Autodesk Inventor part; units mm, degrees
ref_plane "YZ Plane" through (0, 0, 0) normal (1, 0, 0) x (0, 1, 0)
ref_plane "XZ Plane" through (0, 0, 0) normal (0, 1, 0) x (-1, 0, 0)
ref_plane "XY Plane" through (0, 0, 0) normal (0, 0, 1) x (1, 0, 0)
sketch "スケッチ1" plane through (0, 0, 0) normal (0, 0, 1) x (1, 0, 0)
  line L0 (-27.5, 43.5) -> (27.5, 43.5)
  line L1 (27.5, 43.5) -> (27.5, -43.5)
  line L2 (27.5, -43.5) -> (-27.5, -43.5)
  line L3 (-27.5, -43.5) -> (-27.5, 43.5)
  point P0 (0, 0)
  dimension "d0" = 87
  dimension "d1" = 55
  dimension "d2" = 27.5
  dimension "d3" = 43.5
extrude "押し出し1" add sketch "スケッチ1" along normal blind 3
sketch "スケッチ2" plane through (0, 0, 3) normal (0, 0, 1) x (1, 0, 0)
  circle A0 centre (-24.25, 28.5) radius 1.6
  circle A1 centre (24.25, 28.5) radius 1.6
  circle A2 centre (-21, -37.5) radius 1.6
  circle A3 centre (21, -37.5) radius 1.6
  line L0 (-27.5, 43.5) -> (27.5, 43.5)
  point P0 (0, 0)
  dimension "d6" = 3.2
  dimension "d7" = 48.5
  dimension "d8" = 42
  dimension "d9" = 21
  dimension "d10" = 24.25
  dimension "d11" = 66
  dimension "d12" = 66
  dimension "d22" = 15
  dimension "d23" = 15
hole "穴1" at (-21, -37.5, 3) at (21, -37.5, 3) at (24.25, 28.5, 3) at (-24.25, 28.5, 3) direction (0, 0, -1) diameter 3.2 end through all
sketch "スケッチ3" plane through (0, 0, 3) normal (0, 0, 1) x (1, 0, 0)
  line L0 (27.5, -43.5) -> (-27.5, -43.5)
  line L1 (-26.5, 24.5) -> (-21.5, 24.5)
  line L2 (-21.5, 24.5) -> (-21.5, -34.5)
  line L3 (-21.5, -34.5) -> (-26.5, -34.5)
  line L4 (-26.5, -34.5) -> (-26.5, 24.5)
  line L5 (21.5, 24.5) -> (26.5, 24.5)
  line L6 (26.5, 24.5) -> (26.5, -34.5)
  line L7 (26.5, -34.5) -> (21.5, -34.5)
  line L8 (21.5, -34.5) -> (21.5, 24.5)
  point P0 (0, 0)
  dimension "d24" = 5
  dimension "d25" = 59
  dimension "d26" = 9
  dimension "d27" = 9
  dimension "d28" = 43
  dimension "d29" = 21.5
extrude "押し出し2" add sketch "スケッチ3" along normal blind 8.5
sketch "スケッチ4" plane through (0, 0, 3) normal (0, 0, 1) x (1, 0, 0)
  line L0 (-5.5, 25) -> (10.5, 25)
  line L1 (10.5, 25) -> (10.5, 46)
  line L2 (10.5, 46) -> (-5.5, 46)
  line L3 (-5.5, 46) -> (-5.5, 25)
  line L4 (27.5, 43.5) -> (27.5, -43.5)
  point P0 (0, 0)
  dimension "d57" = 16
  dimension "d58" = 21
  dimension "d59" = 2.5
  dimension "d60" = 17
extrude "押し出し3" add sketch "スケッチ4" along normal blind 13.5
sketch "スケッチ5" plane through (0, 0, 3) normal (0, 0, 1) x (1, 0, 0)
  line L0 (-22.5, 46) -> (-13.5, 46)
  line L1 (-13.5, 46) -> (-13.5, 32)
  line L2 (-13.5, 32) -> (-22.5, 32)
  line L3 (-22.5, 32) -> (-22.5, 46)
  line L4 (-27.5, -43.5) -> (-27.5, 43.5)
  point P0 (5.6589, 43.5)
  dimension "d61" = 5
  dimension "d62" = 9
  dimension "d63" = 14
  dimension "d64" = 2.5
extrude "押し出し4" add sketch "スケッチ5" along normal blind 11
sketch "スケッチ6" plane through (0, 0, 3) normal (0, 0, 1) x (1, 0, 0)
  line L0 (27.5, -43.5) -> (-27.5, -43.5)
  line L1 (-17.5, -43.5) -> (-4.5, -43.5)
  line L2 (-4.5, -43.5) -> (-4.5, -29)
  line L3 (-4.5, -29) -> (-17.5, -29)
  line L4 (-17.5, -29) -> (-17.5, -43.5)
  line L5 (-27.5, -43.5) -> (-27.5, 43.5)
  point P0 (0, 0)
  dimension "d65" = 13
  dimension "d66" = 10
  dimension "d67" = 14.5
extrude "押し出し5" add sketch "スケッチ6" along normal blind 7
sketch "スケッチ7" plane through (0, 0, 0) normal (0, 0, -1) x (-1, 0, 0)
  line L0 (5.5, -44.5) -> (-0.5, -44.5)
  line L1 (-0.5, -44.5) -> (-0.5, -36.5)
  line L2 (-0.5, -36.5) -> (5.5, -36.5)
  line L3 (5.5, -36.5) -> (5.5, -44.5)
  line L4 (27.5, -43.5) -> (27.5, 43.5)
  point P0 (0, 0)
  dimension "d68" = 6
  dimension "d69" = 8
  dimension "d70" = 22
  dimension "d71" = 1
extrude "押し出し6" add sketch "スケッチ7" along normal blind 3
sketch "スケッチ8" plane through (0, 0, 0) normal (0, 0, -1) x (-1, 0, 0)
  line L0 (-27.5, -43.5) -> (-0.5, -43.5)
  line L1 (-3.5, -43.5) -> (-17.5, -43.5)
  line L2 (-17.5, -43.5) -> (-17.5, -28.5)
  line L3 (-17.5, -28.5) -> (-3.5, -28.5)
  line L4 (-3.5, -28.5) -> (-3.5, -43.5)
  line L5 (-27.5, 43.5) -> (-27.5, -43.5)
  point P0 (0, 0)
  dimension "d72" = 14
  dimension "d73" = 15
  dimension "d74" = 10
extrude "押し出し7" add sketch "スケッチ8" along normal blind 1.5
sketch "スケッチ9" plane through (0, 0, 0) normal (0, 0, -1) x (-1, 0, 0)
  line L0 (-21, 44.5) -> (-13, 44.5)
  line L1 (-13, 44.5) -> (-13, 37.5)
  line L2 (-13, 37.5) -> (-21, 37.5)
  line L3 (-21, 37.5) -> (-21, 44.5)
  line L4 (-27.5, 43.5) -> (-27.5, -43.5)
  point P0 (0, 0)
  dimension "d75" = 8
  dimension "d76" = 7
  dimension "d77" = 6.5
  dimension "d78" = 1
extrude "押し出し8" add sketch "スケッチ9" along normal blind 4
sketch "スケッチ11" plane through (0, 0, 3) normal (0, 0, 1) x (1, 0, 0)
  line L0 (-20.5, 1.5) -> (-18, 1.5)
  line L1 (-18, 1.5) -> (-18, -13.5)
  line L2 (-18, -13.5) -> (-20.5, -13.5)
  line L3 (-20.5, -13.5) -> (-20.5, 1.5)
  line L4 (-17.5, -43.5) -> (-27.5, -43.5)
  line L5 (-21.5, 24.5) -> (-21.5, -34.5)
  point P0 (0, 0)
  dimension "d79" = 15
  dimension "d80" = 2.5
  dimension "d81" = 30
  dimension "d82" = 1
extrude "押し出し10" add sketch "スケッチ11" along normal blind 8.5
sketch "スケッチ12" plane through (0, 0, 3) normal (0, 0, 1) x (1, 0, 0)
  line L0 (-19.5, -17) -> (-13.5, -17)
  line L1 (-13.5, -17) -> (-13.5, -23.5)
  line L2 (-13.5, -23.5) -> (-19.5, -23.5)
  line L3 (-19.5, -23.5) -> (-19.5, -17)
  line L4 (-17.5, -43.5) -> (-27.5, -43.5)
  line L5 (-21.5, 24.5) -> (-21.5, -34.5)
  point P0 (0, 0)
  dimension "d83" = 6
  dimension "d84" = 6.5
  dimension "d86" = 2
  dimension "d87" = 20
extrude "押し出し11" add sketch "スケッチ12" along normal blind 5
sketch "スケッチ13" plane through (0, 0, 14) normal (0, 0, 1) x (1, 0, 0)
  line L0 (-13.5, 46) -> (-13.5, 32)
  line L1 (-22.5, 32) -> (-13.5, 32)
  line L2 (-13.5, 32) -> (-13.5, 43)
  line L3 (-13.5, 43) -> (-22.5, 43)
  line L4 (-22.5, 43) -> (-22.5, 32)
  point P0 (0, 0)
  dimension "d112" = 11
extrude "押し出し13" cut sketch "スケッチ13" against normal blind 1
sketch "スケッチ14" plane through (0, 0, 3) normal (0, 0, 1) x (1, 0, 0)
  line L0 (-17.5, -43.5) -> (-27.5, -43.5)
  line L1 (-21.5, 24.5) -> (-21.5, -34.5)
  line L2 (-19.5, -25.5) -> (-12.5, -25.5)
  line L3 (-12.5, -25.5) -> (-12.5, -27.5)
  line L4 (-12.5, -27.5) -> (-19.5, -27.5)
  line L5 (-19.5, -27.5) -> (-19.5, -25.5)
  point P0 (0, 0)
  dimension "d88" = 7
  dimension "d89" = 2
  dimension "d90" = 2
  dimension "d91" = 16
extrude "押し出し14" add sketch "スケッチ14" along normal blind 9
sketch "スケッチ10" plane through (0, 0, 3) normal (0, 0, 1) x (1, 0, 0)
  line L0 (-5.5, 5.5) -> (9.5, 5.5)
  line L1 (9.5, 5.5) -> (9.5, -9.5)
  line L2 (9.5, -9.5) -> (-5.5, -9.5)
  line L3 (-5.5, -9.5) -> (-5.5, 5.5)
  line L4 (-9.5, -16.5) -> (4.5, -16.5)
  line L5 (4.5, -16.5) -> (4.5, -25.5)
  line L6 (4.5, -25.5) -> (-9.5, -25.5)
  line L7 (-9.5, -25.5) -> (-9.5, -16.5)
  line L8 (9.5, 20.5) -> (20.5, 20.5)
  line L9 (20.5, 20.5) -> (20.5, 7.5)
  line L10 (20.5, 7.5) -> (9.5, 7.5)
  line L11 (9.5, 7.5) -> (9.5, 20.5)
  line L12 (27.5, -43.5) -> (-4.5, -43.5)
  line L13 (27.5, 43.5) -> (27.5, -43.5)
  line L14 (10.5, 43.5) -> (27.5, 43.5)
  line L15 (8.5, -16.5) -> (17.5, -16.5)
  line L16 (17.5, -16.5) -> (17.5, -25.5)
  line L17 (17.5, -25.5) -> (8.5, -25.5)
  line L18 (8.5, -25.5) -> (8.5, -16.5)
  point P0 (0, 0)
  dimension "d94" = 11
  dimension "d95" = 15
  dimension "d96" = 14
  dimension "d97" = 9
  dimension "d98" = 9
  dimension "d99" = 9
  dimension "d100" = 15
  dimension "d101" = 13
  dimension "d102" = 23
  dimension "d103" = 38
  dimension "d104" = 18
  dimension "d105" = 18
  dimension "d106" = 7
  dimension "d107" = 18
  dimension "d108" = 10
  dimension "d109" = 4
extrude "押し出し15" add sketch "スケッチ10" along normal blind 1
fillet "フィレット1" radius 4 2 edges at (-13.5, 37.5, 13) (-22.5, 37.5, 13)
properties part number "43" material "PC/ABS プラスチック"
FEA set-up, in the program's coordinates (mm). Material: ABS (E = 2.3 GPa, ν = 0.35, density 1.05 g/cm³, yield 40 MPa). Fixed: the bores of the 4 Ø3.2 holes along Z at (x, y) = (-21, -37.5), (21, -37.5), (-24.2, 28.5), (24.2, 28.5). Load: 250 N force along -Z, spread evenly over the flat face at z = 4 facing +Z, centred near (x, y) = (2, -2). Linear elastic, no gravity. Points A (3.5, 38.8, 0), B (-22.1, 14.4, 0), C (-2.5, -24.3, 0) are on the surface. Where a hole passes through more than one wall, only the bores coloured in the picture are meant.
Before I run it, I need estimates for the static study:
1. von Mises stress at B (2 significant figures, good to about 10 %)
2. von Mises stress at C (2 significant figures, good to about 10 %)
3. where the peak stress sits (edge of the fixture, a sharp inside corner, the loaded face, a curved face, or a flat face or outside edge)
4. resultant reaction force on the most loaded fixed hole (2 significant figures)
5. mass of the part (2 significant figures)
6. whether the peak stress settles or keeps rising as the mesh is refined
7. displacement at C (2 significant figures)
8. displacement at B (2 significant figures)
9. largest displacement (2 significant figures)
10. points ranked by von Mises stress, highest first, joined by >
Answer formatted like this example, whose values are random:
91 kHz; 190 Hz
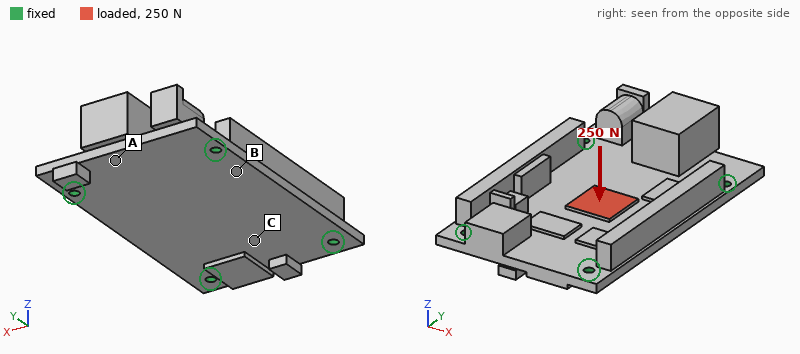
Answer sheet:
3.8 MPa; 5.3 MPa; edge of the fixture; 110 N; 30 g; keeps rising; 0.37 mm; 0.14 mm; 0.81 mm; C > B > A
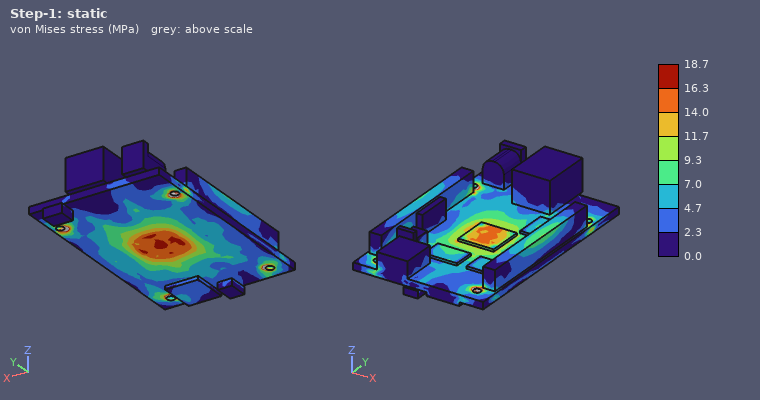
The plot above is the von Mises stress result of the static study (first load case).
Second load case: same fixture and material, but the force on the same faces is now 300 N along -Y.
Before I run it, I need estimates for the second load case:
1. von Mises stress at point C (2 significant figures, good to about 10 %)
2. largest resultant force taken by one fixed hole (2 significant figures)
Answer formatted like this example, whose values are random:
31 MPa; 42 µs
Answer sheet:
1.5 MPa; 85 N
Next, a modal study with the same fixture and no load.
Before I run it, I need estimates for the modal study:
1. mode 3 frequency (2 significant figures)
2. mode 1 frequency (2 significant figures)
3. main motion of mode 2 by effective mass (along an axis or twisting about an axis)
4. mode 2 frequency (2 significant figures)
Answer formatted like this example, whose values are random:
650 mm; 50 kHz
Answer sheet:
1900 Hz; 820 Hz; along Z; 1300 Hz
